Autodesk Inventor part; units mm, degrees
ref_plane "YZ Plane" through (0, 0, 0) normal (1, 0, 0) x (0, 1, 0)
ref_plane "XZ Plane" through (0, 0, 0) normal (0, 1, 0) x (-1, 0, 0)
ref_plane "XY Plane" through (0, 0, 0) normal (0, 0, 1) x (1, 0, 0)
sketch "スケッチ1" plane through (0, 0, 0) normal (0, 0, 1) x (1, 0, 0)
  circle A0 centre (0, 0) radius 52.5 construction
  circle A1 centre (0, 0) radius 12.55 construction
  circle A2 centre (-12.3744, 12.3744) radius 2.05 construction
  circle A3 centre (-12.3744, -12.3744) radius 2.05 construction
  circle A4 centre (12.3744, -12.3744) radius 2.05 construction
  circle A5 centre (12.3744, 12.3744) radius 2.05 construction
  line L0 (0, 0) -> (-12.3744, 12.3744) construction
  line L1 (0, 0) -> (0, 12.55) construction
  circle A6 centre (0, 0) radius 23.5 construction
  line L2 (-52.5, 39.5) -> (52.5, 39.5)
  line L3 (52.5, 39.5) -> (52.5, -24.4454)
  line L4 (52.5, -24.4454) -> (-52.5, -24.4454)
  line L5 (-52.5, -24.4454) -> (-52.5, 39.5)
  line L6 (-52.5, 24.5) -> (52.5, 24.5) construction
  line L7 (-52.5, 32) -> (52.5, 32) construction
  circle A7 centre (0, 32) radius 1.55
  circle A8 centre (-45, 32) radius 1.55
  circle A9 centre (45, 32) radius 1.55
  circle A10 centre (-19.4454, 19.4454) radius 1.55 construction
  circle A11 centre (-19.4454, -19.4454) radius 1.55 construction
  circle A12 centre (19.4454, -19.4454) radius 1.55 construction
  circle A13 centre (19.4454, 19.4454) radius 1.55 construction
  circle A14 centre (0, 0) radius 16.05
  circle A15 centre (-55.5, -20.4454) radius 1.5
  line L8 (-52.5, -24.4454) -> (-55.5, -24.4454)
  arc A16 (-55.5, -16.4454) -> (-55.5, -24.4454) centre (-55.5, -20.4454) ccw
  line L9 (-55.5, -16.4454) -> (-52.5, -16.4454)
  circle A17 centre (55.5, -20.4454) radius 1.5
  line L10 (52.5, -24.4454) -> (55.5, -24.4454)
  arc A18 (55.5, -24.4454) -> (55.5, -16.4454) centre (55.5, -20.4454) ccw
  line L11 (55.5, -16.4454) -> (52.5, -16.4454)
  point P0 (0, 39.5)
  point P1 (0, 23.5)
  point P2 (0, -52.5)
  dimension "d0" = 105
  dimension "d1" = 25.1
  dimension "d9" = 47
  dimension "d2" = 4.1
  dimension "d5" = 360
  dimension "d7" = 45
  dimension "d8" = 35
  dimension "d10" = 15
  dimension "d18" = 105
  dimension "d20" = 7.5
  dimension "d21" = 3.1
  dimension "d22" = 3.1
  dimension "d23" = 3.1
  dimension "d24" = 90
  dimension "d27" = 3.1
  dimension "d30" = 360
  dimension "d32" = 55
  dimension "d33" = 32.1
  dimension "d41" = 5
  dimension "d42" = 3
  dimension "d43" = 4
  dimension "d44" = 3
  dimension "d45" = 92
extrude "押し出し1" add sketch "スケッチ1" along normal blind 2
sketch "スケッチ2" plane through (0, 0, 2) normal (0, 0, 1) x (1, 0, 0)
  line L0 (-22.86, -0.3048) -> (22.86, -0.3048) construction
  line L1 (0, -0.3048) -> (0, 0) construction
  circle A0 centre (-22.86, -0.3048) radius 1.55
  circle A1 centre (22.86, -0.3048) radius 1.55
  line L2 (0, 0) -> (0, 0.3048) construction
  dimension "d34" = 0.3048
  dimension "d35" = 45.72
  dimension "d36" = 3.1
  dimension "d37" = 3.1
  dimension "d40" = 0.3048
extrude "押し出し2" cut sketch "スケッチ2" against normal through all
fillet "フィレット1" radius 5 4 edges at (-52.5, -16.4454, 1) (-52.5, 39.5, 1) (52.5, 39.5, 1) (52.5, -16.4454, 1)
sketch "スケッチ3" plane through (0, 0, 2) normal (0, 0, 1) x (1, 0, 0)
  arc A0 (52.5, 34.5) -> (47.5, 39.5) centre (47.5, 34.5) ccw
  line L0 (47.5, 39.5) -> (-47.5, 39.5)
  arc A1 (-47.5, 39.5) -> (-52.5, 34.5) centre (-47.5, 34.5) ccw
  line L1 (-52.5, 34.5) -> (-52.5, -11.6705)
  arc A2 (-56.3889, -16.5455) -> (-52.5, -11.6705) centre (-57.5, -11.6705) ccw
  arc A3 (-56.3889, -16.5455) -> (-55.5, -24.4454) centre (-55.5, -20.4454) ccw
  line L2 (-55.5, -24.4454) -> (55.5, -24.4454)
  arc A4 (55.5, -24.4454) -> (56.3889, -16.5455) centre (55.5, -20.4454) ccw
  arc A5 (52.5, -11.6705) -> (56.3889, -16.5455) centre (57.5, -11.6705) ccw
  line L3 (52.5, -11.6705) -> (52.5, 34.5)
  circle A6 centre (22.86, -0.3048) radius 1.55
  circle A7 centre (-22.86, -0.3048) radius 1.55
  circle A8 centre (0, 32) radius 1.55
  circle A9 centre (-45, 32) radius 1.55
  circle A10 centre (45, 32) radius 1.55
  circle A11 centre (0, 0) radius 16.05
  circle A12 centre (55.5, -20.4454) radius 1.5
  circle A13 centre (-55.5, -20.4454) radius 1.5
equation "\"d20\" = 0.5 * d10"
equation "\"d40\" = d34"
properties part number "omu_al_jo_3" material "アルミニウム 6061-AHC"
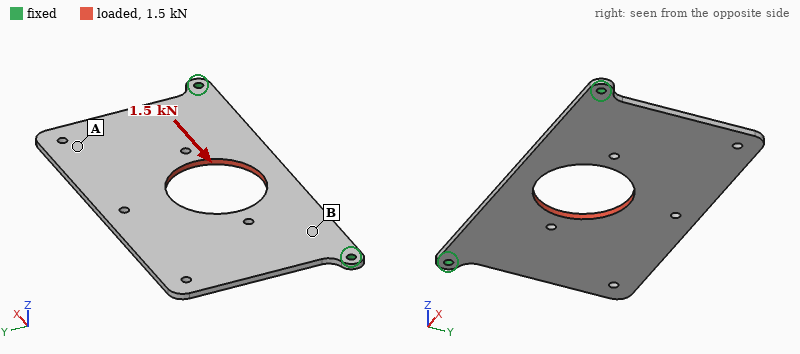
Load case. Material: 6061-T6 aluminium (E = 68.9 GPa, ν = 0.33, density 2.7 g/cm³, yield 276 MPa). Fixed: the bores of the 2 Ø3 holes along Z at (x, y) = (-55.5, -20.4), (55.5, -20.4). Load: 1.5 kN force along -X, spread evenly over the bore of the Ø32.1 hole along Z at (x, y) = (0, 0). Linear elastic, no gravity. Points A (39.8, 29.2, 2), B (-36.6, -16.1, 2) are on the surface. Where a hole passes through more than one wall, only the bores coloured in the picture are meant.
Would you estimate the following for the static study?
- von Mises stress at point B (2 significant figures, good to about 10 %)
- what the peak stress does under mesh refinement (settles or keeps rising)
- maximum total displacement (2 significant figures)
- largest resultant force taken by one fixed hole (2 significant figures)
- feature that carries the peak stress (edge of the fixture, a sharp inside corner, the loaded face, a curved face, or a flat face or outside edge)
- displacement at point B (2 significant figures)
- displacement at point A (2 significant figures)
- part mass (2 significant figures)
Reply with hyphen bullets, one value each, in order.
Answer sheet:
- 18 MPa
- keeps rising
- 26 µm
- 800 N
- edge of the fixture
- 10.0 µm
- 23 µm
- 32 g
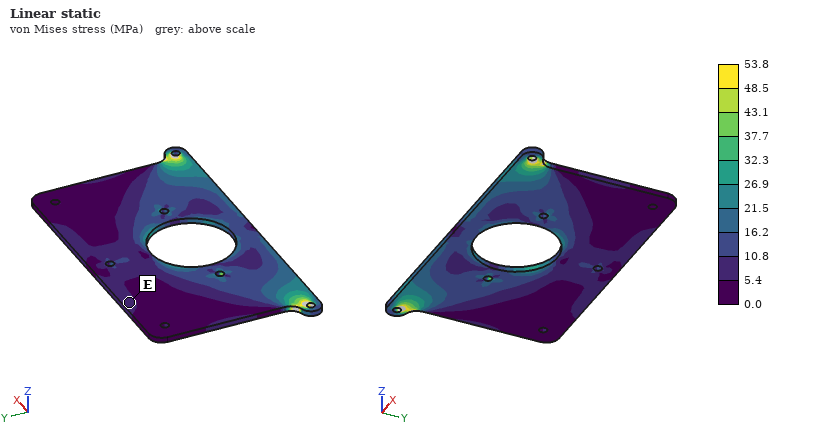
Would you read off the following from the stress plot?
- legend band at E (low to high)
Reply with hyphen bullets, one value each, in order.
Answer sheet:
- 5.4 to 10.8 MPa
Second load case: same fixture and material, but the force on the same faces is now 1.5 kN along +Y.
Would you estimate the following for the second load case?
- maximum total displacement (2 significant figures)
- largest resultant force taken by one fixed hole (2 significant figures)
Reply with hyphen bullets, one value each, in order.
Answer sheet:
- 47 µm
- 890 N
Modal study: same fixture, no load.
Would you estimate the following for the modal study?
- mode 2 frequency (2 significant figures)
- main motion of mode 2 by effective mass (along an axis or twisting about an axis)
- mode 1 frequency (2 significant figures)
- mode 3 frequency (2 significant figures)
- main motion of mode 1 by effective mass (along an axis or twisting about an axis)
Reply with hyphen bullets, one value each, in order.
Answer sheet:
- 640 Hz
- twisting about Y
- 230 Hz
- 840 Hz
- along Z
